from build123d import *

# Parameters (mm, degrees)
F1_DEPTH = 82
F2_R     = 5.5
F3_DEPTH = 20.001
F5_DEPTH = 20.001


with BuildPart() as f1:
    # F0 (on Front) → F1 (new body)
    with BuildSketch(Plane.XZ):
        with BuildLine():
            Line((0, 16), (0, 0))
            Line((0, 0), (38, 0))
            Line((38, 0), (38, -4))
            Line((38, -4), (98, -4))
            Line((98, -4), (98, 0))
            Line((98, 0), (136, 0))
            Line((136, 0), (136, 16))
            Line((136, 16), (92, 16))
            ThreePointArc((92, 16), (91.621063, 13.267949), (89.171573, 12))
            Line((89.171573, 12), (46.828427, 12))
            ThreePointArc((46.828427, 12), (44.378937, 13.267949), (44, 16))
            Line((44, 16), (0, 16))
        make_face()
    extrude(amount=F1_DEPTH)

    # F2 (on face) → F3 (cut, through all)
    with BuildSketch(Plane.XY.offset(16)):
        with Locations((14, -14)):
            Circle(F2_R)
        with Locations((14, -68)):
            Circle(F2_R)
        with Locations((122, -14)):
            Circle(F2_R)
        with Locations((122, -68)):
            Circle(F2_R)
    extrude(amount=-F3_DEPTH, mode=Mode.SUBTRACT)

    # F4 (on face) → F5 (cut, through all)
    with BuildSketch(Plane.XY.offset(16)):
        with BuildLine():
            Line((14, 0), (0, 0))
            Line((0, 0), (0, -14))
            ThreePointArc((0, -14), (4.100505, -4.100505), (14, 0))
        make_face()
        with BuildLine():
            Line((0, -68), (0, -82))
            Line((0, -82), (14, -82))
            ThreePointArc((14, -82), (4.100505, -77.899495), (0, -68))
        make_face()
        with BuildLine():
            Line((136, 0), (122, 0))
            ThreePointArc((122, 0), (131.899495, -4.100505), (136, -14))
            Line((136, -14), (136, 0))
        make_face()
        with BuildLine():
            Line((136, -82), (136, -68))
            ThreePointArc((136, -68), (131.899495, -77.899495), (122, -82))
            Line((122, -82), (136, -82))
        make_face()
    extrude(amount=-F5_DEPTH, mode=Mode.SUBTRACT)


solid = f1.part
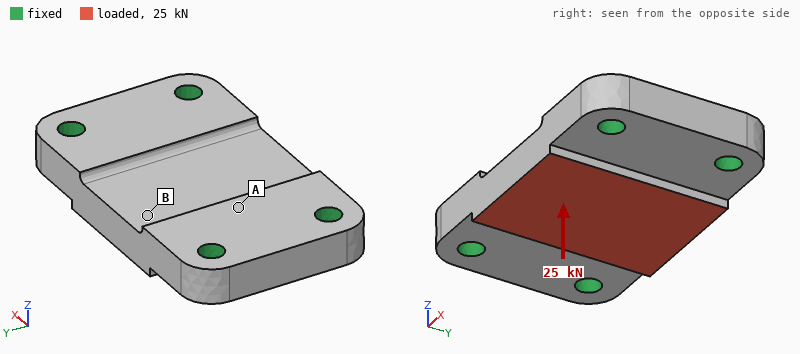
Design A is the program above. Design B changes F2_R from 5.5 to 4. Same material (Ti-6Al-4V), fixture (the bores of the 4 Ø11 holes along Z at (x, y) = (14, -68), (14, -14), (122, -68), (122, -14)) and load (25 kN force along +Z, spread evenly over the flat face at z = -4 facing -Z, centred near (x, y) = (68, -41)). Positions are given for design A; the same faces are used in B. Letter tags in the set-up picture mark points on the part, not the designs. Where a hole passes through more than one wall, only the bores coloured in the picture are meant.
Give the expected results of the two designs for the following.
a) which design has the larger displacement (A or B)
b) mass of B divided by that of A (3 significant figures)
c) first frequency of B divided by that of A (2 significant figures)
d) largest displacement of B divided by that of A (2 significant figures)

B
1.02
0.92
1.2
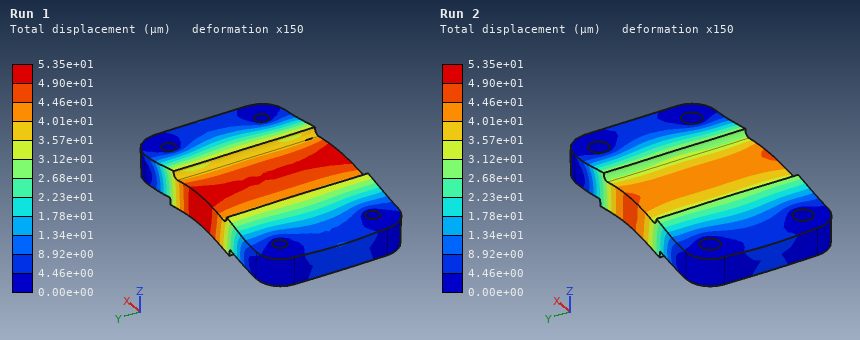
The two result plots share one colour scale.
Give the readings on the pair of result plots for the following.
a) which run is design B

Run 1
